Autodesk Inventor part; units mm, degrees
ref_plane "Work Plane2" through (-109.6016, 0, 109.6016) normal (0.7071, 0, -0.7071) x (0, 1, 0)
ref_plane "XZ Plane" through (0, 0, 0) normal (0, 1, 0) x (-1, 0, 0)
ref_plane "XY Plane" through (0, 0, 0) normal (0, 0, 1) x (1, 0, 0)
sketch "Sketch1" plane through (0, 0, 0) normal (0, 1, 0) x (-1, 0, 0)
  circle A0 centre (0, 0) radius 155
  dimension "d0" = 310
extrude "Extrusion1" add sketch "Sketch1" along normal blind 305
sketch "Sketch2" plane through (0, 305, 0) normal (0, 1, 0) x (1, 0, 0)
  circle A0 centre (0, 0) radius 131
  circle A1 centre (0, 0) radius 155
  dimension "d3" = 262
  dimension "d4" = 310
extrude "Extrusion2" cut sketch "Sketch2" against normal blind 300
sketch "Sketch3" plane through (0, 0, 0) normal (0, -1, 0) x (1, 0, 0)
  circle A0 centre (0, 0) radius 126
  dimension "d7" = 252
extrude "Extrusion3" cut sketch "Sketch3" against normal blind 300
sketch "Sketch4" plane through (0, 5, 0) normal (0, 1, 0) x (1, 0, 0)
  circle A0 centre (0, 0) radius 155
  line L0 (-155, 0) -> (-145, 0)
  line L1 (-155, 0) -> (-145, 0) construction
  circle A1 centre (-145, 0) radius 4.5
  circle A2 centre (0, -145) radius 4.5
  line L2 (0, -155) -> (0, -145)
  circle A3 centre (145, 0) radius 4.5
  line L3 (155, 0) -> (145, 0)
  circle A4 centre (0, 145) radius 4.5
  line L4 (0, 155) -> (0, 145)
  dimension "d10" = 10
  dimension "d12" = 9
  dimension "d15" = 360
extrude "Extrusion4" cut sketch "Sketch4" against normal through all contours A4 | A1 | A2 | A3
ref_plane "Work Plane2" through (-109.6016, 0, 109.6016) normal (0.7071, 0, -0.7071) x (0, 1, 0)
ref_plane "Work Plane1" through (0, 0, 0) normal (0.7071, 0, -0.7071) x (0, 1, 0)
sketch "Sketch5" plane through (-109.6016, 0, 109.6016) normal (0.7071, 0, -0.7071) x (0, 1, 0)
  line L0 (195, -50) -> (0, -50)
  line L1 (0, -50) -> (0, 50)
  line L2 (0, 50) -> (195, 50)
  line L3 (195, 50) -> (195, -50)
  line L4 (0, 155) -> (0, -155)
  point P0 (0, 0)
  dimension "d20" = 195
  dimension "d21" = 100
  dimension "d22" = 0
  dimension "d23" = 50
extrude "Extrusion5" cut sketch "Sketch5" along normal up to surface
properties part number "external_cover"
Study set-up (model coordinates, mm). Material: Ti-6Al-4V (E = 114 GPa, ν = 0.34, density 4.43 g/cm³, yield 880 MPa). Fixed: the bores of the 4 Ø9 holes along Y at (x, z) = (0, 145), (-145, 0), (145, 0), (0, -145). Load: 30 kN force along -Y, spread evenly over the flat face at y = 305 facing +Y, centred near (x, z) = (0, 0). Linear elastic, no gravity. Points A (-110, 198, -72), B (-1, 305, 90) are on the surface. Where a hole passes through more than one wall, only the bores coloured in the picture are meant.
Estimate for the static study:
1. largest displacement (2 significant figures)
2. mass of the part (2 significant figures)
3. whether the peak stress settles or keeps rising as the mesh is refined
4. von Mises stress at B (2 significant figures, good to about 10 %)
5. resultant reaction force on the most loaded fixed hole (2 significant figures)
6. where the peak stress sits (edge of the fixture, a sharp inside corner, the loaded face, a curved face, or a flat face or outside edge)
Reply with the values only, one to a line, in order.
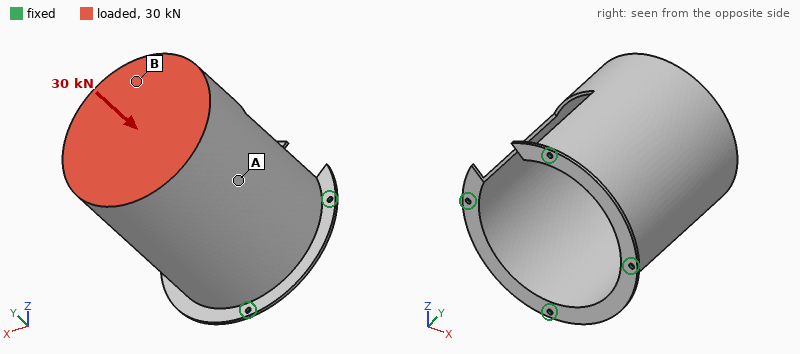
2.3 mm
6.5 kg
keeps rising
83 MPa
7.6 kN
edge of the fixture
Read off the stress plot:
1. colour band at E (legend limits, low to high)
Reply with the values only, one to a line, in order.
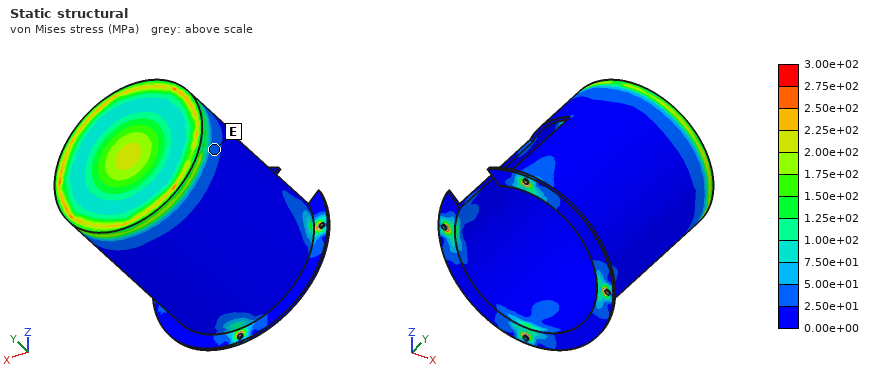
2.50e+01 to 5.00e+01 MPa
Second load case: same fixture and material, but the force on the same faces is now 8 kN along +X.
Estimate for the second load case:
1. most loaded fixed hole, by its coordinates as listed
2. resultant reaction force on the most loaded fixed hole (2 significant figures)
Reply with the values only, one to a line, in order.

(145, 0)
11 kN
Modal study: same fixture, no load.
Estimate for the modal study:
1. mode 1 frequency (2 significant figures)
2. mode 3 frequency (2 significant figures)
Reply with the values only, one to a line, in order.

290 Hz
620 Hz
